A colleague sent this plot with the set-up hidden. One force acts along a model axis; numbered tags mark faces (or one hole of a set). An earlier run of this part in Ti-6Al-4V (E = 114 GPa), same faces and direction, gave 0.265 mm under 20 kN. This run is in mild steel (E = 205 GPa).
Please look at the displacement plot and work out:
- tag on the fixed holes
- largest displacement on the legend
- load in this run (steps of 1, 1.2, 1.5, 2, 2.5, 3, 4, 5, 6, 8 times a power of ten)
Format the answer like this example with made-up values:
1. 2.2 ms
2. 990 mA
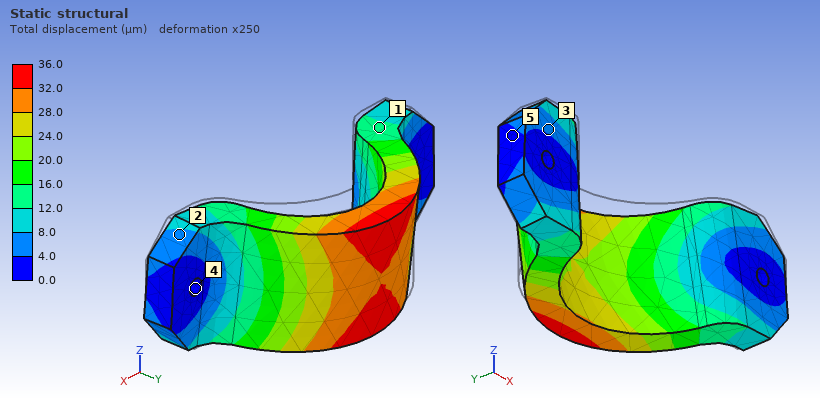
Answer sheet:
1. 4
2. 36.0 µm
3. 5 kN
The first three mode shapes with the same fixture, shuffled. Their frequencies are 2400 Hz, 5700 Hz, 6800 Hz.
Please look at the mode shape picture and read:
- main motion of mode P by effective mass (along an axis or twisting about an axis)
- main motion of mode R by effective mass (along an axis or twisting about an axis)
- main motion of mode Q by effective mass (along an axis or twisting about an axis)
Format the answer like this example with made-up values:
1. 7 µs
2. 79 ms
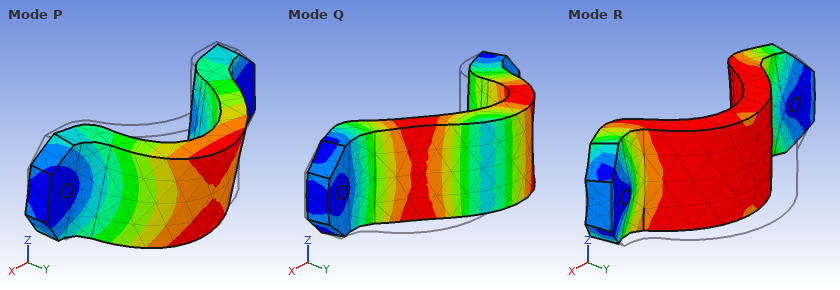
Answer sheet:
1. along Z
2. along Y
3. along X
